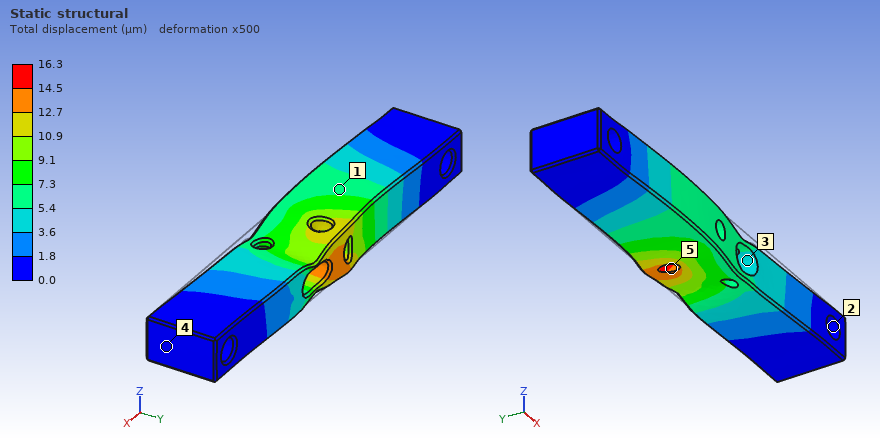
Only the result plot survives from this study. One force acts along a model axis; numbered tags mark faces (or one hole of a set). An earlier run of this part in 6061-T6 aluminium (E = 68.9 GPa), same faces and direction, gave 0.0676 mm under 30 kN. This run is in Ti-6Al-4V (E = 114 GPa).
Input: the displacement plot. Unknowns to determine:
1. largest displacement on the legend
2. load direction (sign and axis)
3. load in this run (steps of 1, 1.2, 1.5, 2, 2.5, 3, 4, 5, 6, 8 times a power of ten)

16.3 µm
-X
12 kN
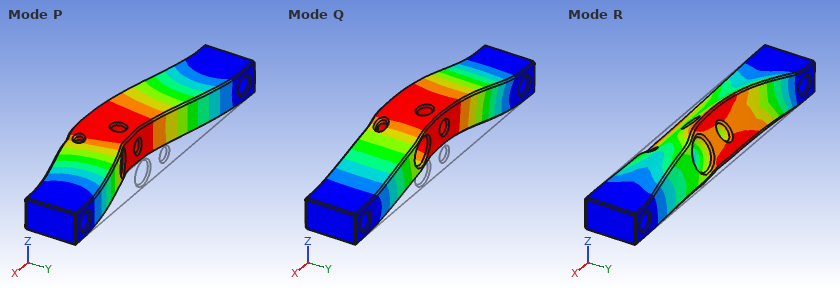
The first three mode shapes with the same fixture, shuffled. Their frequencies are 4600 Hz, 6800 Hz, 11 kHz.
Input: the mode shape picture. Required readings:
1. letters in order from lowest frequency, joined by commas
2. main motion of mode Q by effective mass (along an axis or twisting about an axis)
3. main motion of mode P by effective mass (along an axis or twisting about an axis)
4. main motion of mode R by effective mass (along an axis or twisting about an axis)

Q, P, R
along Z
along Y
twisting about X
